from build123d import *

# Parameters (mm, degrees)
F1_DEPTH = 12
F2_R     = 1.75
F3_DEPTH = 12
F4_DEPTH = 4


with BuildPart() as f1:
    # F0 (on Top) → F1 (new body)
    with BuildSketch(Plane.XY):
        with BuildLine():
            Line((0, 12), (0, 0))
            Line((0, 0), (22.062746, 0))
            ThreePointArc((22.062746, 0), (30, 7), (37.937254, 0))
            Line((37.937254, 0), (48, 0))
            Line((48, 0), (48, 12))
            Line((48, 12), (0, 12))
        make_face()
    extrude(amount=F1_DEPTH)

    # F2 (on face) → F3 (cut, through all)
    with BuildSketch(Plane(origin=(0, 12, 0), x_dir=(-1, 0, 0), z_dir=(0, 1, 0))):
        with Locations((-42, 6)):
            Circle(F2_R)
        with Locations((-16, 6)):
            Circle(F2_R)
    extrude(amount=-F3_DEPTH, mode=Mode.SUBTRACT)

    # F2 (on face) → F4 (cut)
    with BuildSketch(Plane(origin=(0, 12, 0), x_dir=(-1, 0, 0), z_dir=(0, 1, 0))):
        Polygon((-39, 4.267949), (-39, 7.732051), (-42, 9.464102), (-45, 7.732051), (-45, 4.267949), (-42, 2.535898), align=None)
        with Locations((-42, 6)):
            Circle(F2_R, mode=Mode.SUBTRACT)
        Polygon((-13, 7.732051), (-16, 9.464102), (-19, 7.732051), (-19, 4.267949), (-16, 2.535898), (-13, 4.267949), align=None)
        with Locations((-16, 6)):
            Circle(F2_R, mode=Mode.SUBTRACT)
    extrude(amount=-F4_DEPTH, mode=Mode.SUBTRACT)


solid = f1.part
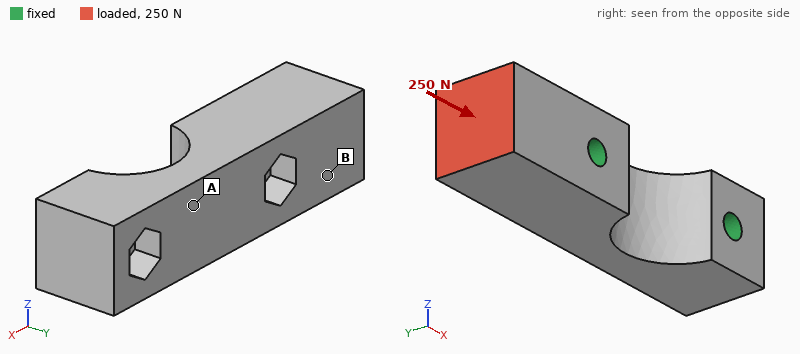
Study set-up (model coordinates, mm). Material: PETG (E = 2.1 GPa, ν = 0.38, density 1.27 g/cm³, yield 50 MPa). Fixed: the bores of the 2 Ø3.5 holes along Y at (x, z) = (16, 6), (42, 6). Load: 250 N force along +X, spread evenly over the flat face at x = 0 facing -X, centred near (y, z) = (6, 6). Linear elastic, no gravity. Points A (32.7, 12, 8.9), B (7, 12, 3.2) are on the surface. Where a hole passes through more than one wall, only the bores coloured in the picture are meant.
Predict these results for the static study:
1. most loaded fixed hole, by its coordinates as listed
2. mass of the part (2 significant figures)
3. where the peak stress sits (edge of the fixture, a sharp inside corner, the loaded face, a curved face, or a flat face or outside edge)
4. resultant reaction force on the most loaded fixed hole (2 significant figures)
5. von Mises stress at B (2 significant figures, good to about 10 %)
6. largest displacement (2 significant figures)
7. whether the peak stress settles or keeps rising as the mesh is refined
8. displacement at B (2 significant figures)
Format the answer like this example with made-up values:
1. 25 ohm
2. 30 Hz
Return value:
1. (16, 6)
2. 7.0 g
3. edge of the fixture
4. 230 N
5. 1.6 MPa
6. 30 µm
7. keeps rising
8. 21 µm
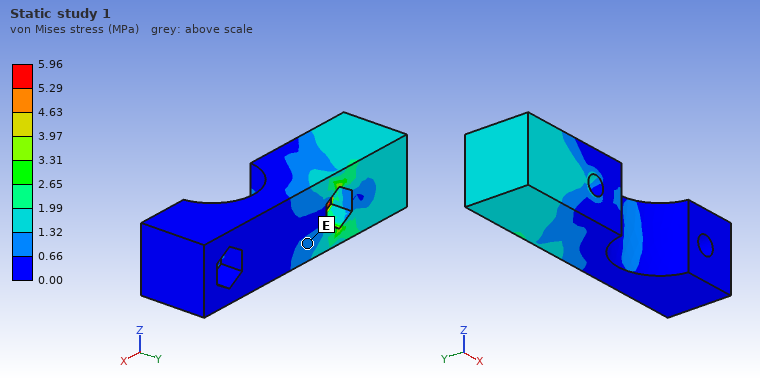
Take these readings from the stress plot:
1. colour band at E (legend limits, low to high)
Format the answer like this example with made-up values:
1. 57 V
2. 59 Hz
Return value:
1. 0.66 to 1.32 MPa
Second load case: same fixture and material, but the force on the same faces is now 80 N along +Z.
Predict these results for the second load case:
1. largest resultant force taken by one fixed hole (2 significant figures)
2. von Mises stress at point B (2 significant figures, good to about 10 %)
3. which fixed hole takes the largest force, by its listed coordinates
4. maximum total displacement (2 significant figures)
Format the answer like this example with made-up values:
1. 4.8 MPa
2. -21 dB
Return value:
1. 100 N
2. 1.5 MPa
3. (16, 6)
4. 95 µm
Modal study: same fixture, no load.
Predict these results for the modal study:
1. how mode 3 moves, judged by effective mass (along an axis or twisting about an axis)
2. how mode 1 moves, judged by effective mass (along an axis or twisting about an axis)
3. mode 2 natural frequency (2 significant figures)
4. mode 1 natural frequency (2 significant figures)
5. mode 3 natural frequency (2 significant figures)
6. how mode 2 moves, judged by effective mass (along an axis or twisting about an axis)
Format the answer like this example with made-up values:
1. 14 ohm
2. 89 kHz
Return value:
1. along Z
2. along Z
3. 5400 Hz
4. 4800 Hz
5. 8100 Hz
6. along Y
